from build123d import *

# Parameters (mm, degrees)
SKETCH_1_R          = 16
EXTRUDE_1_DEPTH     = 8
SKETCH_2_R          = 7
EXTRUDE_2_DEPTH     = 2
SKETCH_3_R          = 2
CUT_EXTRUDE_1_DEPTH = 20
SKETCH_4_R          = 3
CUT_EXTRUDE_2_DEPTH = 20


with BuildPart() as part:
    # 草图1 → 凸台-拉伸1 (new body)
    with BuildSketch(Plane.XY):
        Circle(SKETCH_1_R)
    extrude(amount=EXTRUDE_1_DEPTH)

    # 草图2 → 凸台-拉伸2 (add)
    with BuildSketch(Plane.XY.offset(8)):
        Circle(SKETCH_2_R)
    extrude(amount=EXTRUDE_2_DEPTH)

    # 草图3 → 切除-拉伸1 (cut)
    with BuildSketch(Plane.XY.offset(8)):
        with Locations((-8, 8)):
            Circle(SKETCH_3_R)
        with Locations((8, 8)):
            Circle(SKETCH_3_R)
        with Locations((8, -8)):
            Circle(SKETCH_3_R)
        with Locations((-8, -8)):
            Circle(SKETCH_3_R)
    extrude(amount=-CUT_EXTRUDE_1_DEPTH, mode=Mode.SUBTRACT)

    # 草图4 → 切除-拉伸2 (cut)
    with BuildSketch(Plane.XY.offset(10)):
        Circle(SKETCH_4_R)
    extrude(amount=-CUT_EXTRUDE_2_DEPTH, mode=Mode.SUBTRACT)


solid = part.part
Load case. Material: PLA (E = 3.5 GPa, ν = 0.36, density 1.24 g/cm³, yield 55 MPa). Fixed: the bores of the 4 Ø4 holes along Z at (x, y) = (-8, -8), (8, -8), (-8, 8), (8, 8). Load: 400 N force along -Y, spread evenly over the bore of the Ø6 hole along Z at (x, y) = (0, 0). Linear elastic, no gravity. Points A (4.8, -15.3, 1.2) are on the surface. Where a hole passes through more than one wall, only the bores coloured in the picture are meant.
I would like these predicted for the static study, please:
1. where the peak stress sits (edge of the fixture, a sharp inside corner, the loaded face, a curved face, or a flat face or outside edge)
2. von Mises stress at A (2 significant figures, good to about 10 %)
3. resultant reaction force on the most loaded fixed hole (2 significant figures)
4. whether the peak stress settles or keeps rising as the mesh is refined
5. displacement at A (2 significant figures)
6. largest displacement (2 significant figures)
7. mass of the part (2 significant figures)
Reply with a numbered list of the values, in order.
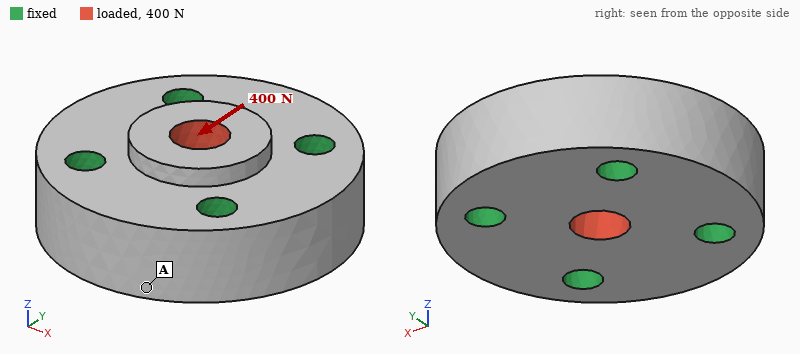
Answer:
1. edge of the fixture
2. 0.52 MPa
3. 110 N
4. keeps rising
5. 1.5 µm
6. 7.7 µm
7. 7.5 g
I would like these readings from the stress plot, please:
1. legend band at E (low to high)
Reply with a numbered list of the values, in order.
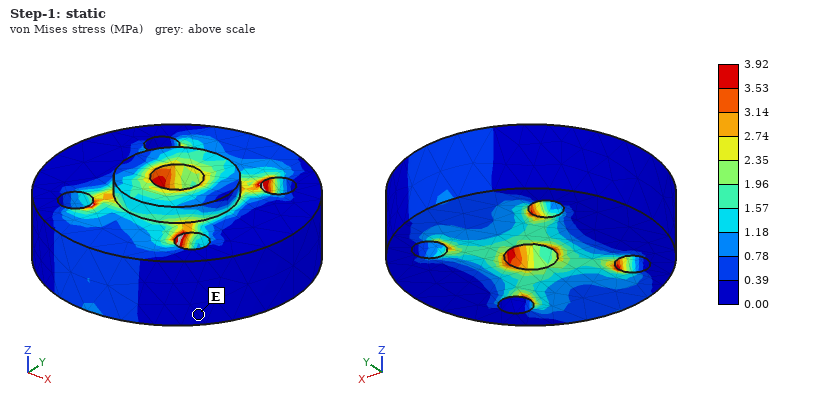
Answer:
1. 0.00 to 0.39 MPa
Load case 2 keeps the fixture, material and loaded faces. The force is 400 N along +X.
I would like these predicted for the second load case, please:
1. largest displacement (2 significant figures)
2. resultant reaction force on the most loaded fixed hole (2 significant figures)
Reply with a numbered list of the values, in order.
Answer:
1. 7.7 µm
2. 110 N
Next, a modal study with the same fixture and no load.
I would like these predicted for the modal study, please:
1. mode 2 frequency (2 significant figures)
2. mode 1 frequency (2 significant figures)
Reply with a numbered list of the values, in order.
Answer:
1. 23 kHz
2. 22 kHz
